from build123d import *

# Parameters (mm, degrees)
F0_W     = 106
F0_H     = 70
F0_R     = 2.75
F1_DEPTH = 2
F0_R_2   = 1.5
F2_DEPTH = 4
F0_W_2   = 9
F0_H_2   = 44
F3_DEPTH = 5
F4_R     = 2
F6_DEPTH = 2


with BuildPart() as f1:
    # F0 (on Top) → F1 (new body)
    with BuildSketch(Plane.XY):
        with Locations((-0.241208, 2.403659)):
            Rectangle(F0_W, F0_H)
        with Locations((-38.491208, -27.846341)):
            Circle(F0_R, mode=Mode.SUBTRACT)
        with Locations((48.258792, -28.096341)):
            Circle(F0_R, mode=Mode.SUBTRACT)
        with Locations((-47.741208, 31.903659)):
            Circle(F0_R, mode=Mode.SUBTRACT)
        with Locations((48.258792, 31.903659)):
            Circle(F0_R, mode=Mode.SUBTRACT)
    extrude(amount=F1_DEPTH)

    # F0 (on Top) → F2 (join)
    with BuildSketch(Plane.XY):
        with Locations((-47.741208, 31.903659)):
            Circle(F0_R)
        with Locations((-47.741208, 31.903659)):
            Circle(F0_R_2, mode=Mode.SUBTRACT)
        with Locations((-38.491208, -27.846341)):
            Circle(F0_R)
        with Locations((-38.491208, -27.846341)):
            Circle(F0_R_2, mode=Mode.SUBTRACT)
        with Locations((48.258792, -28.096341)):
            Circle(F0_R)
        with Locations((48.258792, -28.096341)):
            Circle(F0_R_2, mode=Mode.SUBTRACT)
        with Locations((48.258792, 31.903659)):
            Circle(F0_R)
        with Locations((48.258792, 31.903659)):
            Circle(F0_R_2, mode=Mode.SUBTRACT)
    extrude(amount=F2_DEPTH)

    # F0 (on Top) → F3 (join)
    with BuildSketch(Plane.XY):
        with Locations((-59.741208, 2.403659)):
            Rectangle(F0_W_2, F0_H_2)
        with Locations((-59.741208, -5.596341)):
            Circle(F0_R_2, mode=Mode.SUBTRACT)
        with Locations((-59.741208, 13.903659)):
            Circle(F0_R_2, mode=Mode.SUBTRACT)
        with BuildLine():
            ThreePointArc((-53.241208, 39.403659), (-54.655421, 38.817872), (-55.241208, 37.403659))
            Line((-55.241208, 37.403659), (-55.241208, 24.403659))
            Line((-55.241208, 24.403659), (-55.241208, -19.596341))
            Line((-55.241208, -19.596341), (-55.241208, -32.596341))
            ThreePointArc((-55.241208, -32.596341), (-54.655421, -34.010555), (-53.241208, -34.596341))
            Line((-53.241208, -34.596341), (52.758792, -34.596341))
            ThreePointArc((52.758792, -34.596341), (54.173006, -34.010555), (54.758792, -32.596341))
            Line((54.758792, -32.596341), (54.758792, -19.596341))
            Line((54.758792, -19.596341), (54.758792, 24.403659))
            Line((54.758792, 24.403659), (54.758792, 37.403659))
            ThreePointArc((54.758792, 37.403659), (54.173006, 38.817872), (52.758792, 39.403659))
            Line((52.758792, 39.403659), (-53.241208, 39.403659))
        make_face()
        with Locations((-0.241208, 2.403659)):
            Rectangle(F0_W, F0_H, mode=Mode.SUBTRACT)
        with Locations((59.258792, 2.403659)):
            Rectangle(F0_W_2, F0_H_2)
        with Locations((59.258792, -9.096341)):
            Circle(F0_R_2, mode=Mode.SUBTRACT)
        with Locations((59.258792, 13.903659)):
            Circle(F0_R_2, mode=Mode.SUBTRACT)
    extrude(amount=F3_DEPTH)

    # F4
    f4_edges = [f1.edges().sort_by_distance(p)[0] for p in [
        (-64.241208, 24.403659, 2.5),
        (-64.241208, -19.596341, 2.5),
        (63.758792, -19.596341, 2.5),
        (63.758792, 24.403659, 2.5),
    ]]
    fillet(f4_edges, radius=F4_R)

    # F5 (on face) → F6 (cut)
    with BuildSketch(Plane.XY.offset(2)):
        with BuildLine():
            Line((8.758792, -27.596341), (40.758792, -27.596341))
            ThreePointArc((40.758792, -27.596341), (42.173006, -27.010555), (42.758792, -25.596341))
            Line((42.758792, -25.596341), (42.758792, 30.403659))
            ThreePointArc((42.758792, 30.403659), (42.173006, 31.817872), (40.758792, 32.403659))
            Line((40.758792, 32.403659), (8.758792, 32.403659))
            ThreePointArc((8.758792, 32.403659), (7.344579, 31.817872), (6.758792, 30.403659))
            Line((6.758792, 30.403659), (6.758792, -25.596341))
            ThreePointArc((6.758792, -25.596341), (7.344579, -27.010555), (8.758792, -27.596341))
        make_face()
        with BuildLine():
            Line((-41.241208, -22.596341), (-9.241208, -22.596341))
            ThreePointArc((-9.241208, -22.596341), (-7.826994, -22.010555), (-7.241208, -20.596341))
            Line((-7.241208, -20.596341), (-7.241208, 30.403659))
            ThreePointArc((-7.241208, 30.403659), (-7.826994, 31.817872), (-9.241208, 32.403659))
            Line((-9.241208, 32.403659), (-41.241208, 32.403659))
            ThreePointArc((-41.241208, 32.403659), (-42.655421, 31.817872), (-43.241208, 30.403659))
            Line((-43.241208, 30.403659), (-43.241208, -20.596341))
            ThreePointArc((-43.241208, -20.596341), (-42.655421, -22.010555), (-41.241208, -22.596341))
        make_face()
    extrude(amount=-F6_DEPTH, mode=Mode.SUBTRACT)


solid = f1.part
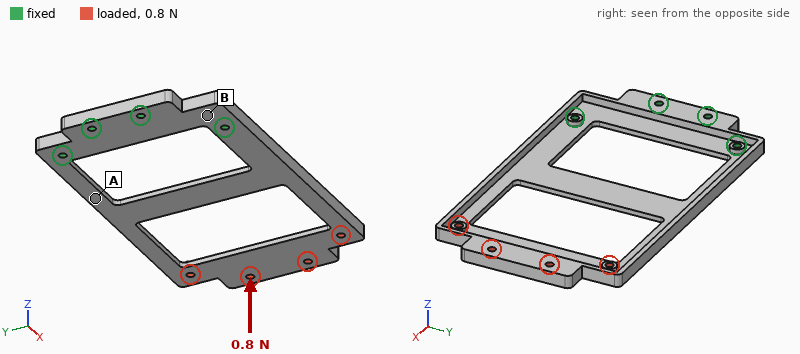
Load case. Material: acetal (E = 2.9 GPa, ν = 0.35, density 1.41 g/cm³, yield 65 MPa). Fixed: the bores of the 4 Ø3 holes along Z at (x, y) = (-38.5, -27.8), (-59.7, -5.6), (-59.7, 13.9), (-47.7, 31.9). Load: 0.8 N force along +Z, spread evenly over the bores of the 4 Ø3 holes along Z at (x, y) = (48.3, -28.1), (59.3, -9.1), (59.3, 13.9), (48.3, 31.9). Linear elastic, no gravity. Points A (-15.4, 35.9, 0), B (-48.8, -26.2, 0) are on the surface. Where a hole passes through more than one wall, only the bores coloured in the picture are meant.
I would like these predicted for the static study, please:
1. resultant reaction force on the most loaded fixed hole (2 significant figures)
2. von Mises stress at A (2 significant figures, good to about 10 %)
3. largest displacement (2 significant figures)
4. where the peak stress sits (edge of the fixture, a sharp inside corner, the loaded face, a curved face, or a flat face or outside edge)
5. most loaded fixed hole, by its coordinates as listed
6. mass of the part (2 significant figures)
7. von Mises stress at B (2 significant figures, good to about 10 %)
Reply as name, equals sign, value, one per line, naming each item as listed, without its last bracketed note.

resultant reaction force on the most loaded fixed hole = 1.9 N
von Mises stress at A = 1.1 MPa
largest displacement = 1.6 mm
where the peak stress sits = a curved face
most loaded fixed hole, by its coordinates as listed = (-38.5, -27.8)
mass of the part = 20 g
von Mises stress at B = 0.36 MPa
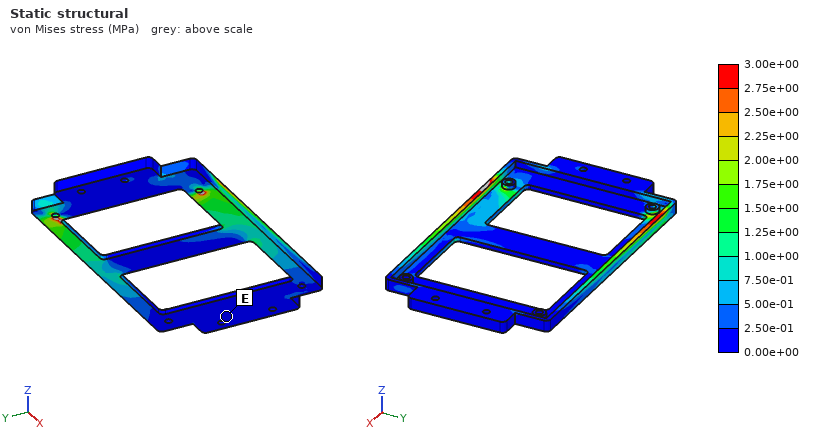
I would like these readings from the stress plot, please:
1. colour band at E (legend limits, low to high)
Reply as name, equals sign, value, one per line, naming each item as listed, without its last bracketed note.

colour band at E = 0.00e+00 to 2.50e-01 MPa
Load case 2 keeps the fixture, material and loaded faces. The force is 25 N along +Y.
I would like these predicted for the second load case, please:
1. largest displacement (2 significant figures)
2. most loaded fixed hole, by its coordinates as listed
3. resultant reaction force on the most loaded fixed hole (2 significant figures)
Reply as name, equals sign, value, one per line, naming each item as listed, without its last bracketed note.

largest displacement = 1.5 mm
most loaded fixed hole, by its coordinates as listed = (-38.5, -27.8)
resultant reaction force on the most loaded fixed hole = 47 N
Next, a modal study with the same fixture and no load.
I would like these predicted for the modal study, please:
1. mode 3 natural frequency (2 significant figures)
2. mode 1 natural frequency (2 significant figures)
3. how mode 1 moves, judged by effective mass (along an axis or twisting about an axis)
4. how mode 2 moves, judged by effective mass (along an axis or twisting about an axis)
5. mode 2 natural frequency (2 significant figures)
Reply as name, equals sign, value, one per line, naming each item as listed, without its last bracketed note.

mode 3 natural frequency = 290 Hz
mode 1 natural frequency = 47 Hz
how mode 1 moves, judged by effective mass = along Z
how mode 2 moves, judged by effective mass = twisting about X
mode 2 natural frequency = 130 Hz
